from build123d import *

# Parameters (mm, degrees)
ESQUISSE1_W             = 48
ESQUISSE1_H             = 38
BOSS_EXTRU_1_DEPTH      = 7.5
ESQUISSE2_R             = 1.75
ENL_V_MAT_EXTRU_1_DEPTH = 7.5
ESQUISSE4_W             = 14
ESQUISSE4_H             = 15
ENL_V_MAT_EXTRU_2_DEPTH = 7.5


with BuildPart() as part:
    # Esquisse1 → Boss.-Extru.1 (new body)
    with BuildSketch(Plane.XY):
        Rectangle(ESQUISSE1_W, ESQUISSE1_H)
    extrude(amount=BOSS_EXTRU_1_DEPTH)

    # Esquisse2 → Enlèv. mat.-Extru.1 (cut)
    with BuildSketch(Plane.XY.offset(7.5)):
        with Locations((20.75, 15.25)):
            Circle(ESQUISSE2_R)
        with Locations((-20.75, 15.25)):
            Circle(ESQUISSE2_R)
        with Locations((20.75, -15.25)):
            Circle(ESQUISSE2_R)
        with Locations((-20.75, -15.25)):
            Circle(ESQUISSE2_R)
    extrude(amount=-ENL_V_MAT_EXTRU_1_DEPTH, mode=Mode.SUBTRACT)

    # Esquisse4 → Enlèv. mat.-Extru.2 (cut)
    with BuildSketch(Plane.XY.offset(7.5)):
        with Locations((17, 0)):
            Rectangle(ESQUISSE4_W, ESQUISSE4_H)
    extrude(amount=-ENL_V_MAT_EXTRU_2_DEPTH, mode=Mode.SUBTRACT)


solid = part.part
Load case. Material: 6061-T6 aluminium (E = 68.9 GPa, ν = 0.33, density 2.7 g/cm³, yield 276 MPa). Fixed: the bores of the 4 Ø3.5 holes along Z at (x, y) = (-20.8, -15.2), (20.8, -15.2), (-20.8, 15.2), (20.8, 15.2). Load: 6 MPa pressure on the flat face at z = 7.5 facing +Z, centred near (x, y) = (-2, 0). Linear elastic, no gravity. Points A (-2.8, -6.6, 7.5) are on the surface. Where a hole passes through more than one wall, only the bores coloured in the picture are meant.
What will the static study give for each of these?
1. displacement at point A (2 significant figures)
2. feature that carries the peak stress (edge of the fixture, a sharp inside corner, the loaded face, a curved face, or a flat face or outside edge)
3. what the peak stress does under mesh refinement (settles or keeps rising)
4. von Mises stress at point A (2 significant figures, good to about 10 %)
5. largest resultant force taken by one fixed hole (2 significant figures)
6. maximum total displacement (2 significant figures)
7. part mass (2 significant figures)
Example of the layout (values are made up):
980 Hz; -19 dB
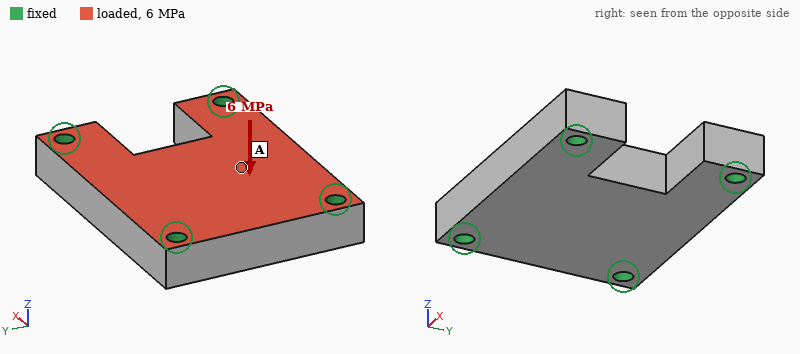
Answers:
39 µm; edge of the fixture; keeps rising; 40 MPa; 2.6 kN; 42 µm; 32 g
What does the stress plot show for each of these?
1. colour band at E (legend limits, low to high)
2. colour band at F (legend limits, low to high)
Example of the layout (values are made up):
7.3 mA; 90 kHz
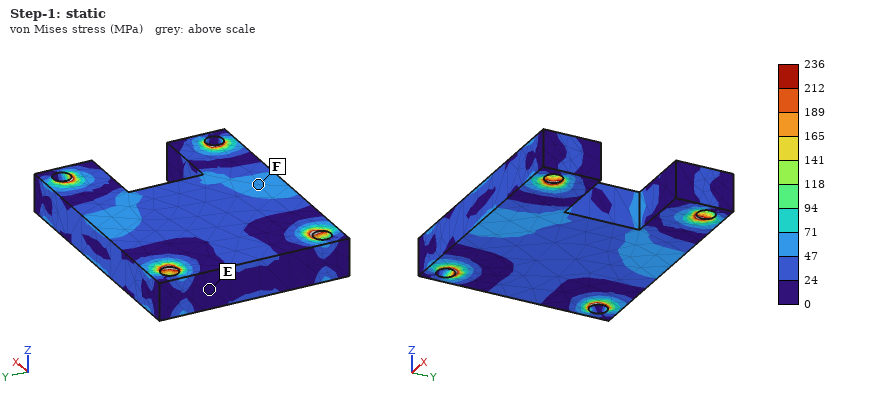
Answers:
0 to 24 MPa; 47 to 71 MPa
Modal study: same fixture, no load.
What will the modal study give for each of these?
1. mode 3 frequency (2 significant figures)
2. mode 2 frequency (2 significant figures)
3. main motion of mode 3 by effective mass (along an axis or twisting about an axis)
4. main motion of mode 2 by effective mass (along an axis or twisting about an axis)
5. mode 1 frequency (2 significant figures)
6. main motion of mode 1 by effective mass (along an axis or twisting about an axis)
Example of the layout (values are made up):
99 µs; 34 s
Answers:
25 kHz; 22 kHz; along Y; twisting about X; 15 kHz; along Z
